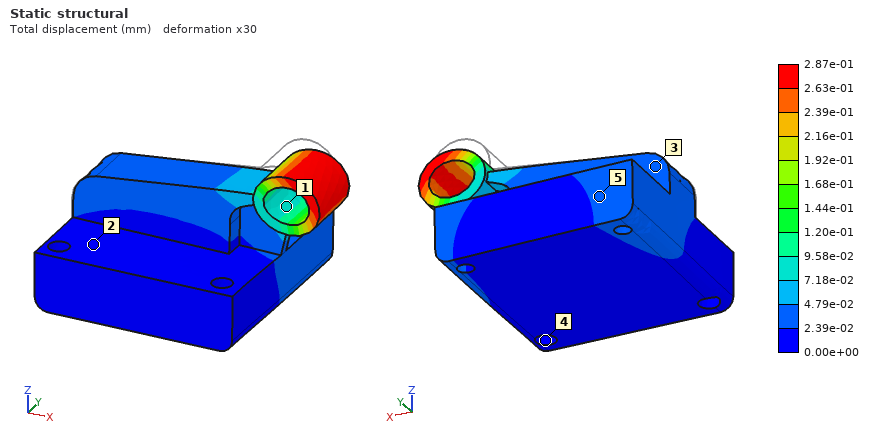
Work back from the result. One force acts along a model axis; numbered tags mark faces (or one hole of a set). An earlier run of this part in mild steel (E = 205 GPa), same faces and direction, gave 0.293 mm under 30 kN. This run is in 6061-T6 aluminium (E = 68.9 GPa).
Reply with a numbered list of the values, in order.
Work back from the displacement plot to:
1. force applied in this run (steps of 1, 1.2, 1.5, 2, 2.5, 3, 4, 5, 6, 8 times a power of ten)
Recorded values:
1. 10 kN
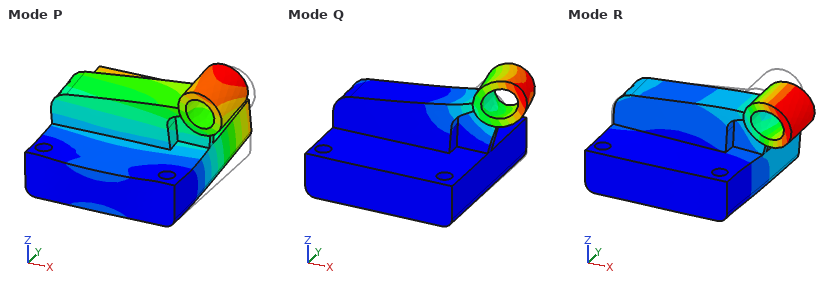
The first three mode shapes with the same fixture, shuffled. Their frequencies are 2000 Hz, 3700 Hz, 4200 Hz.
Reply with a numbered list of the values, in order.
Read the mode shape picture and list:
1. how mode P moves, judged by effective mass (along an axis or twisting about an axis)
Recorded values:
1. along Z
